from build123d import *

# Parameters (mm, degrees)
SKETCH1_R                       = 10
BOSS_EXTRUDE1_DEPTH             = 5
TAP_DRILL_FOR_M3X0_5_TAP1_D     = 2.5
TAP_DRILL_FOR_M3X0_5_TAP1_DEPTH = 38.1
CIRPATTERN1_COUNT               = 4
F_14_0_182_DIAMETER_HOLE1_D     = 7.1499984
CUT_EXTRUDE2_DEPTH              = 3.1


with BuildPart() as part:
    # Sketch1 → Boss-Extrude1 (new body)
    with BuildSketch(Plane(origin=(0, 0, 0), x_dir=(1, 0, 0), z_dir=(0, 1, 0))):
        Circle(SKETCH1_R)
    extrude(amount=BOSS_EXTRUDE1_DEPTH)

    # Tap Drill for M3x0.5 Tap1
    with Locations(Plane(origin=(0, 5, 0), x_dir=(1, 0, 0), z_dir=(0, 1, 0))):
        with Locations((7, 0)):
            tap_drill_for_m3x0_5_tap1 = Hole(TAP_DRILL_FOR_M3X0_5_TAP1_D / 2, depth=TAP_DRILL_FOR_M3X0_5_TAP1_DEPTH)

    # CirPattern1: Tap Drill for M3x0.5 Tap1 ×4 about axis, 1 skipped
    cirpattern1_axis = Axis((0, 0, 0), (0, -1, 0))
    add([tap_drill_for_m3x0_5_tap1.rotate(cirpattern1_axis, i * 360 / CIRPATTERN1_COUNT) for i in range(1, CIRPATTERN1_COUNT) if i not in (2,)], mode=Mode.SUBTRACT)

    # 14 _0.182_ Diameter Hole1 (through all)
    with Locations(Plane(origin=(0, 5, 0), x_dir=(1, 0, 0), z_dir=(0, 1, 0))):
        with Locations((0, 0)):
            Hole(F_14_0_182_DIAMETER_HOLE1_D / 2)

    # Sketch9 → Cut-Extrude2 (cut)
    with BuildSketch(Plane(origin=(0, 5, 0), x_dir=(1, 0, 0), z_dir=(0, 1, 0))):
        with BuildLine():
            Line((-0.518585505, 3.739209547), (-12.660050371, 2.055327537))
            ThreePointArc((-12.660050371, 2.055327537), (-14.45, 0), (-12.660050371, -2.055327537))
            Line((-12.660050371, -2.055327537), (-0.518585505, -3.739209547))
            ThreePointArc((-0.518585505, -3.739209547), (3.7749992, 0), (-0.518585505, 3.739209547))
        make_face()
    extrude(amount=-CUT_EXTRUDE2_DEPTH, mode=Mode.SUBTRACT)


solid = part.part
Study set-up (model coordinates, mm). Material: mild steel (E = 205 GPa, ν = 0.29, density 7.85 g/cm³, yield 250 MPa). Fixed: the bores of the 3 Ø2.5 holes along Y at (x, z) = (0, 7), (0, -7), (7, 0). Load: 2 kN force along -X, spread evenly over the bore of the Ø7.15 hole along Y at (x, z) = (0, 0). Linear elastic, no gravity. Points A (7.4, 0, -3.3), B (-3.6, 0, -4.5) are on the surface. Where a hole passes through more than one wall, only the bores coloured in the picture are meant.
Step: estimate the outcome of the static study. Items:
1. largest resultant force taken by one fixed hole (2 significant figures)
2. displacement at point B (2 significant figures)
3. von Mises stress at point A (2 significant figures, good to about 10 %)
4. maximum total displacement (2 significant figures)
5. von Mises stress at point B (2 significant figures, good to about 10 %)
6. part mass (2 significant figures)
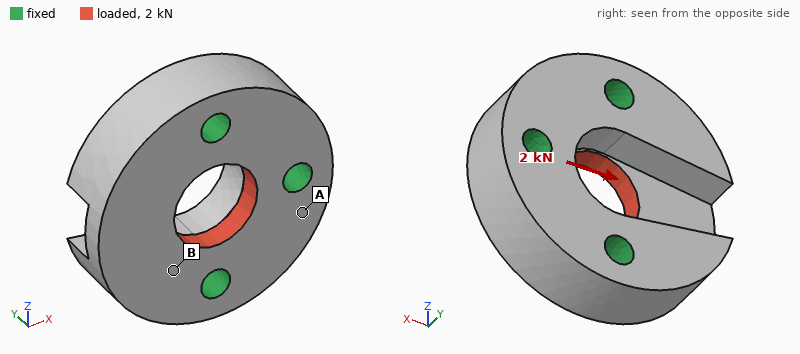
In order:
710 N
1.2 µm
17 MPa
3.3 µm
46 MPa
9.1 g
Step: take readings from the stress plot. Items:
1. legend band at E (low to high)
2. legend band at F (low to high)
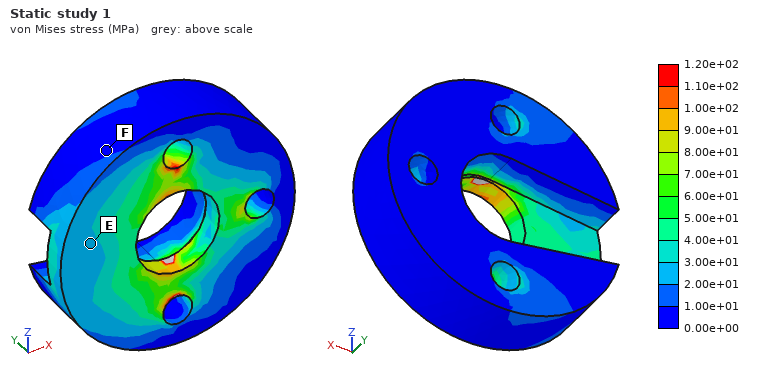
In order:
2.00e+01 to 3.00e+01 MPa
0.00e+00 to 1.00e+01 MPa
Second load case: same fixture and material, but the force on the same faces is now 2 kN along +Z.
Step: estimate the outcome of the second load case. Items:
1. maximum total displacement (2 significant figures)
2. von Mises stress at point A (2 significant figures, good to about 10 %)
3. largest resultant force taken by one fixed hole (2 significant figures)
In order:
2.2 µm
12 MPa
810 N
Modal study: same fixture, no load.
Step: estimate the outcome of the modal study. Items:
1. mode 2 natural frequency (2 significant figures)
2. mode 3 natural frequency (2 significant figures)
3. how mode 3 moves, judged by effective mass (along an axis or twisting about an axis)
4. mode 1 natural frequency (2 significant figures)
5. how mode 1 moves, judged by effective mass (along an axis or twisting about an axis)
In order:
60 kHz
71 kHz
along Z
42 kHz
along Y
